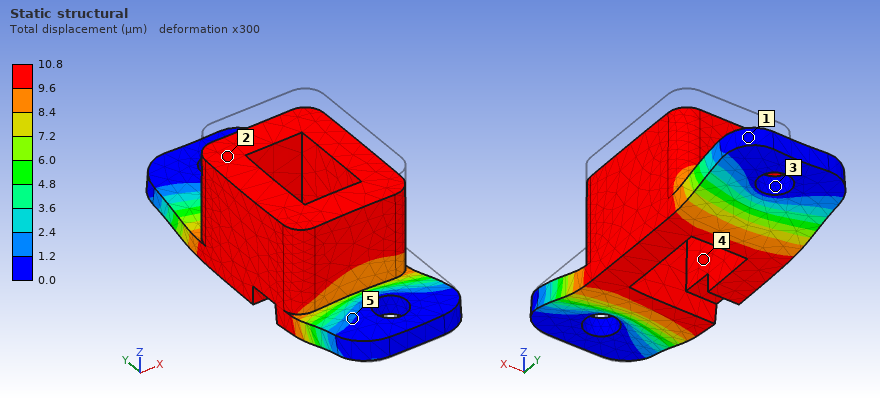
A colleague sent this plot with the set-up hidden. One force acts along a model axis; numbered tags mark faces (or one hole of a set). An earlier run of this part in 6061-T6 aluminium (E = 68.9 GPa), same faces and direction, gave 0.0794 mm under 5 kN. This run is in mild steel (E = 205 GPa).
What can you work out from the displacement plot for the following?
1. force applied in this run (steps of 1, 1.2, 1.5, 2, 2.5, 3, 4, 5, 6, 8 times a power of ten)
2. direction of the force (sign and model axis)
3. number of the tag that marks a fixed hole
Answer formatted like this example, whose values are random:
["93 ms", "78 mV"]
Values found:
["2 kN", "-Z", "3"]
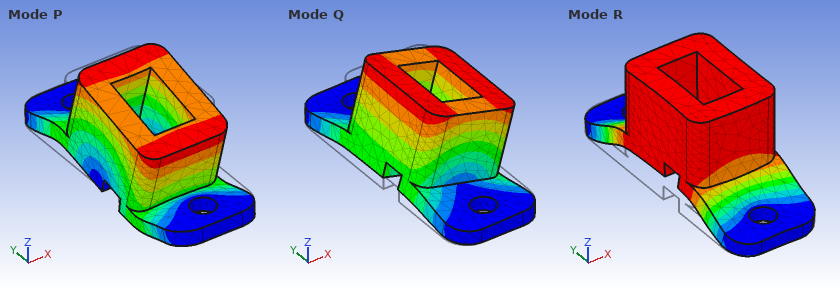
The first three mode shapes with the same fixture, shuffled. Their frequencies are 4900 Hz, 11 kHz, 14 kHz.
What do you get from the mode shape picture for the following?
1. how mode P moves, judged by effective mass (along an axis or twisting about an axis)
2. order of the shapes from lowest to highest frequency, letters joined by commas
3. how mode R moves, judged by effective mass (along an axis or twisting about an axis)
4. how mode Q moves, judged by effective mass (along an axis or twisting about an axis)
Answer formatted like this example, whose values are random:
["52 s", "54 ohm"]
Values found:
["along Y", "Q, R, P", "along Z", "along X"]
